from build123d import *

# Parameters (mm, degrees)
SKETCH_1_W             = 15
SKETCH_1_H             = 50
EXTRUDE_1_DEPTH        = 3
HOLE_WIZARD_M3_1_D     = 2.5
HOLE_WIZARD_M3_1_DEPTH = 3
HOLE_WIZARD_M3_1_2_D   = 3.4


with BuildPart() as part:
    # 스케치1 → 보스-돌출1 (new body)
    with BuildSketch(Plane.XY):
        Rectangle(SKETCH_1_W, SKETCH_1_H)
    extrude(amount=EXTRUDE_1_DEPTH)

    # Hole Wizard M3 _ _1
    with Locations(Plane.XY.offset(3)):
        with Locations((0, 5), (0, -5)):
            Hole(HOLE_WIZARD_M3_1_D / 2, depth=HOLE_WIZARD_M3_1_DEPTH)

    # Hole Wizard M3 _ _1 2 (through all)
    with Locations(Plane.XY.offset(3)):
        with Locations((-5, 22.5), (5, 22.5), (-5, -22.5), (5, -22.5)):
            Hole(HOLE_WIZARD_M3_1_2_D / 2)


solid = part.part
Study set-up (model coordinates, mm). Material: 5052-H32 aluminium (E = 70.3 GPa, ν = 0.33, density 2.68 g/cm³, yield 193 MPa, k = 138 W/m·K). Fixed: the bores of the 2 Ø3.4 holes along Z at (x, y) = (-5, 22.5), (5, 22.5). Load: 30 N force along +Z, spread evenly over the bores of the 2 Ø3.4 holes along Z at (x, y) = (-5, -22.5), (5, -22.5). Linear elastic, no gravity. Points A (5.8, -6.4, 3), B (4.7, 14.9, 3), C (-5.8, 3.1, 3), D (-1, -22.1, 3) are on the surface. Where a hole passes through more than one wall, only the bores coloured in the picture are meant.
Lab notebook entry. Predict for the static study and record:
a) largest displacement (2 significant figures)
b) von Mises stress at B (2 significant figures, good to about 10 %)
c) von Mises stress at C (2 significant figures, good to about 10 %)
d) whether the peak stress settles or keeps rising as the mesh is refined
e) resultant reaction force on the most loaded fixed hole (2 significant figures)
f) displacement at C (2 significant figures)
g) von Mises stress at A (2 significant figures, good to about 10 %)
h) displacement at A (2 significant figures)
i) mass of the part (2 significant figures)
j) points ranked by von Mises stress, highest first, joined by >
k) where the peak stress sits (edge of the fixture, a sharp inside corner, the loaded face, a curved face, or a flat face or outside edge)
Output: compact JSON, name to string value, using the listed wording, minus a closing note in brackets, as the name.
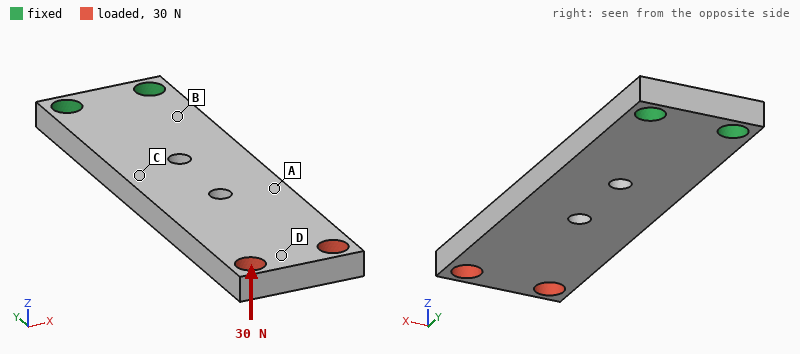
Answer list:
{"largest displacement": "0.40 mm", "von Mises stress at B": "49 MPa", "von Mises stress at C": "37 MPa", "whether the peak stress settles or keeps rising as the mesh is refined": "keeps rising", "resultant reaction force on the most loaded fixed hole": "15 N", "displacement at C": "0.082 mm", "von Mises stress at A": "24 MPa", "displacement at A": "0.17 mm", "mass of the part": "5.7 g", "points ranked by von Mises stress, highest first, joined by >": "B > C > A > D", "where the peak stress sits": "edge of the fixture"}
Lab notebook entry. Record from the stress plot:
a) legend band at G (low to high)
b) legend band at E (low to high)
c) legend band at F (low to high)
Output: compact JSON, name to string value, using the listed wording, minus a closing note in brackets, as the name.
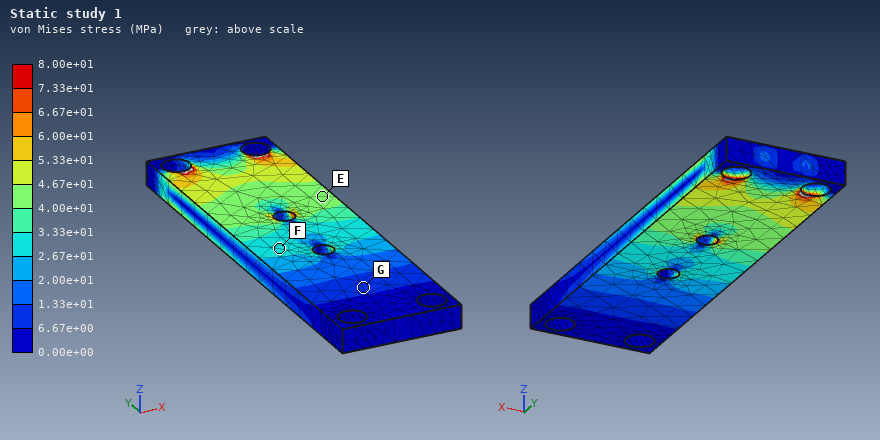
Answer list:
{"legend band at G": "6.67e+00 to 1.33e+01 MPa", "legend band at E": "4.00e+01 to 4.67e+01 MPa", "legend band at F": "2.67e+01 to 3.33e+01 MPa"}
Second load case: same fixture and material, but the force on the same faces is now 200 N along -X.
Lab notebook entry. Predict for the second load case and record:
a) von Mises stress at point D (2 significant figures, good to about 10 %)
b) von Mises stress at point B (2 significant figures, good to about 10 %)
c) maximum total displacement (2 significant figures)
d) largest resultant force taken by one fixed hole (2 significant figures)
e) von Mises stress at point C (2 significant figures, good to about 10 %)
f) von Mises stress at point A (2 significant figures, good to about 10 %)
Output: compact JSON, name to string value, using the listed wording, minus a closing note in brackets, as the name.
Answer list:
{"von Mises stress at point D": "9.1 MPa", "von Mises stress at point B": "43 MPa", "maximum total displacement": "0.12 mm", "largest resultant force taken by one fixed hole": "810 N", "von Mises stress at point C": "35 MPa", "von Mises stress at point A": "22 MPa"}
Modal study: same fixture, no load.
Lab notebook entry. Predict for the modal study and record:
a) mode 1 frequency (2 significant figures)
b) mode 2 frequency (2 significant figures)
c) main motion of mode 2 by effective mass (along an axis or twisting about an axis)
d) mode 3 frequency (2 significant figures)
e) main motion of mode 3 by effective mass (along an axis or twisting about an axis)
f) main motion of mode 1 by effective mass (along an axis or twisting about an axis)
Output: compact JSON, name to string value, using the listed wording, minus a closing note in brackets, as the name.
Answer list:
{"mode 1 frequency": "1200 Hz", "mode 2 frequency": "5600 Hz", "main motion of mode 2 by effective mass": "along X", "mode 3 frequency": "6800 Hz", "main motion of mode 3 by effective mass": "twisting about Y", "main motion of mode 1 by effective mass": "along Z"}
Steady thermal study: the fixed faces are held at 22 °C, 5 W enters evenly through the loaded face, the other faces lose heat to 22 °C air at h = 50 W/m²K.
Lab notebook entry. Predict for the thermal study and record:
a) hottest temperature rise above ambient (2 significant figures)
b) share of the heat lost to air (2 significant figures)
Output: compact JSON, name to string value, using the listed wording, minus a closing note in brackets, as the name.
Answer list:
{"hottest temperature rise above ambient": "33 K", "share of the heat lost to air": "26 %"}
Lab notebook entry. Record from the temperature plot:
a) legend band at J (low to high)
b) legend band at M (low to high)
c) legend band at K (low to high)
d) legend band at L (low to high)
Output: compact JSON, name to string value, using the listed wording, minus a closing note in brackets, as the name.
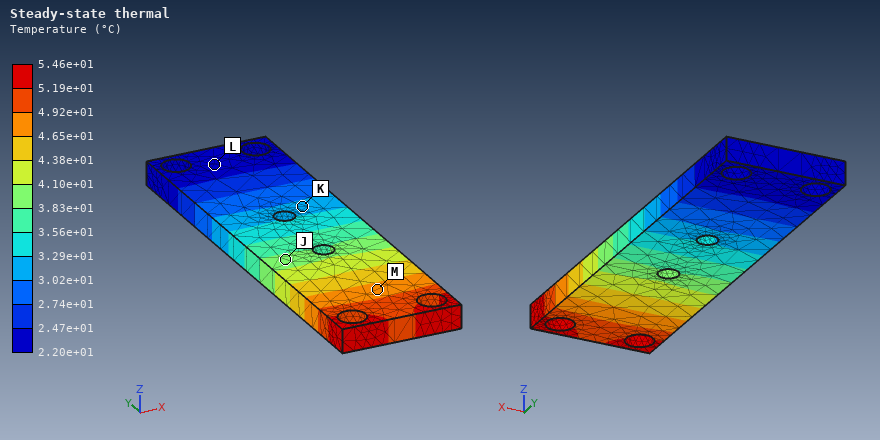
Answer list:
{"legend band at J": "3.83e+01 to 4.10e+01 °C", "legend band at M": "4.65e+01 to 4.92e+01 °C", "legend band at K": "3.02e+01 to 3.29e+01 °C", "legend band at L": "2.20e+01 to 2.47e+01 °C"}
